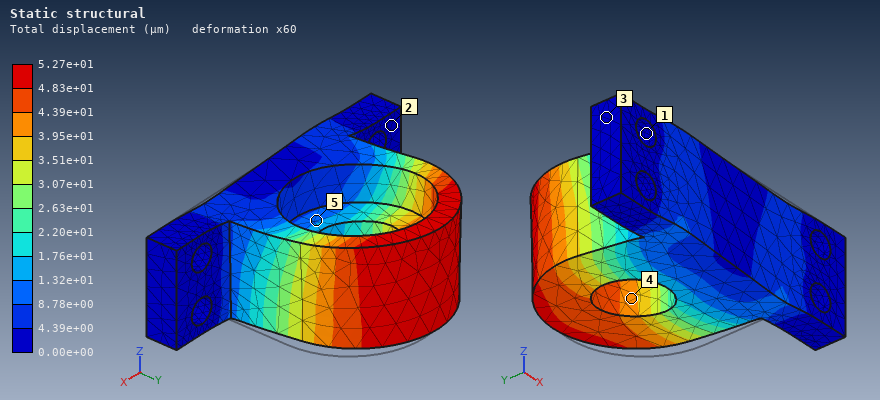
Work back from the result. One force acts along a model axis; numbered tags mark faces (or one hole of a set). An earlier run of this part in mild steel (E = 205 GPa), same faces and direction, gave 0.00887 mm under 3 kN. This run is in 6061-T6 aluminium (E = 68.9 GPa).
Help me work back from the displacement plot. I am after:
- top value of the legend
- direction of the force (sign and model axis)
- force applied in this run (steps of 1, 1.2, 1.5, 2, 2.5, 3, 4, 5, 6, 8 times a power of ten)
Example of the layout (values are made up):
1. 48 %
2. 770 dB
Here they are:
1. 5.27e+01 µm
2. -X
3. 6 kN
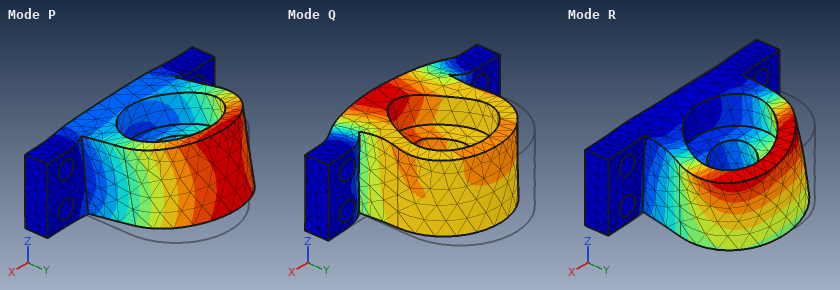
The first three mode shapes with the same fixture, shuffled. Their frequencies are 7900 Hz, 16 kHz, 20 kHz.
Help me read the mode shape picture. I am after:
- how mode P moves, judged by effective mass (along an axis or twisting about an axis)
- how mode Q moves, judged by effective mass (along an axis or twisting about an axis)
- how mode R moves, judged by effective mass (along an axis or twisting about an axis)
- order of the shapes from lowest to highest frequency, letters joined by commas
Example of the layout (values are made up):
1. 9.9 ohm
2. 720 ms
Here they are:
1. along Z
2. along Y
3. along X
4. P, R, Q
